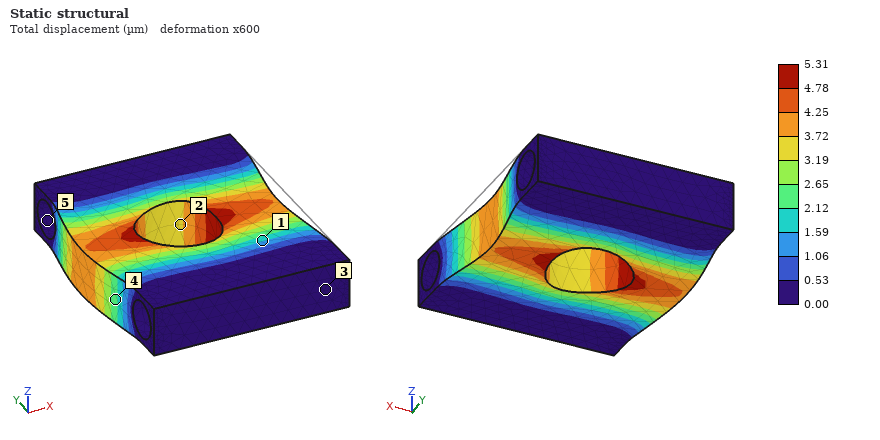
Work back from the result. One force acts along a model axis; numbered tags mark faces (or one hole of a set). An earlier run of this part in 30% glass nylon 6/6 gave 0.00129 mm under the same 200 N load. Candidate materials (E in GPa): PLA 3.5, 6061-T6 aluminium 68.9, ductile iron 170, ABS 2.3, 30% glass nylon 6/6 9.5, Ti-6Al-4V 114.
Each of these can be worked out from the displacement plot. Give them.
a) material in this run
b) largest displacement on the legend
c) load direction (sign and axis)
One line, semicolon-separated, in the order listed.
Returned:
ABS; 5.31 µm; -X
